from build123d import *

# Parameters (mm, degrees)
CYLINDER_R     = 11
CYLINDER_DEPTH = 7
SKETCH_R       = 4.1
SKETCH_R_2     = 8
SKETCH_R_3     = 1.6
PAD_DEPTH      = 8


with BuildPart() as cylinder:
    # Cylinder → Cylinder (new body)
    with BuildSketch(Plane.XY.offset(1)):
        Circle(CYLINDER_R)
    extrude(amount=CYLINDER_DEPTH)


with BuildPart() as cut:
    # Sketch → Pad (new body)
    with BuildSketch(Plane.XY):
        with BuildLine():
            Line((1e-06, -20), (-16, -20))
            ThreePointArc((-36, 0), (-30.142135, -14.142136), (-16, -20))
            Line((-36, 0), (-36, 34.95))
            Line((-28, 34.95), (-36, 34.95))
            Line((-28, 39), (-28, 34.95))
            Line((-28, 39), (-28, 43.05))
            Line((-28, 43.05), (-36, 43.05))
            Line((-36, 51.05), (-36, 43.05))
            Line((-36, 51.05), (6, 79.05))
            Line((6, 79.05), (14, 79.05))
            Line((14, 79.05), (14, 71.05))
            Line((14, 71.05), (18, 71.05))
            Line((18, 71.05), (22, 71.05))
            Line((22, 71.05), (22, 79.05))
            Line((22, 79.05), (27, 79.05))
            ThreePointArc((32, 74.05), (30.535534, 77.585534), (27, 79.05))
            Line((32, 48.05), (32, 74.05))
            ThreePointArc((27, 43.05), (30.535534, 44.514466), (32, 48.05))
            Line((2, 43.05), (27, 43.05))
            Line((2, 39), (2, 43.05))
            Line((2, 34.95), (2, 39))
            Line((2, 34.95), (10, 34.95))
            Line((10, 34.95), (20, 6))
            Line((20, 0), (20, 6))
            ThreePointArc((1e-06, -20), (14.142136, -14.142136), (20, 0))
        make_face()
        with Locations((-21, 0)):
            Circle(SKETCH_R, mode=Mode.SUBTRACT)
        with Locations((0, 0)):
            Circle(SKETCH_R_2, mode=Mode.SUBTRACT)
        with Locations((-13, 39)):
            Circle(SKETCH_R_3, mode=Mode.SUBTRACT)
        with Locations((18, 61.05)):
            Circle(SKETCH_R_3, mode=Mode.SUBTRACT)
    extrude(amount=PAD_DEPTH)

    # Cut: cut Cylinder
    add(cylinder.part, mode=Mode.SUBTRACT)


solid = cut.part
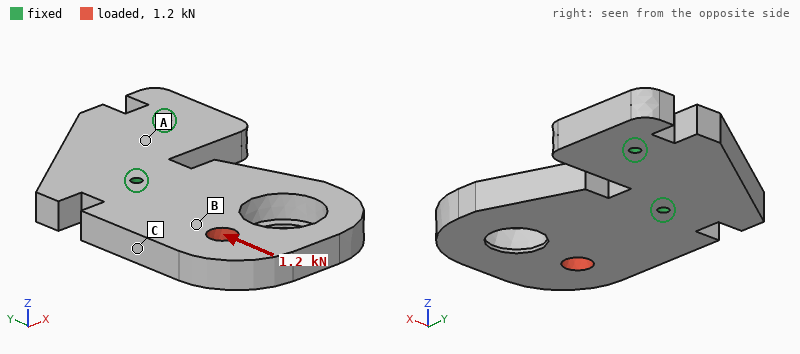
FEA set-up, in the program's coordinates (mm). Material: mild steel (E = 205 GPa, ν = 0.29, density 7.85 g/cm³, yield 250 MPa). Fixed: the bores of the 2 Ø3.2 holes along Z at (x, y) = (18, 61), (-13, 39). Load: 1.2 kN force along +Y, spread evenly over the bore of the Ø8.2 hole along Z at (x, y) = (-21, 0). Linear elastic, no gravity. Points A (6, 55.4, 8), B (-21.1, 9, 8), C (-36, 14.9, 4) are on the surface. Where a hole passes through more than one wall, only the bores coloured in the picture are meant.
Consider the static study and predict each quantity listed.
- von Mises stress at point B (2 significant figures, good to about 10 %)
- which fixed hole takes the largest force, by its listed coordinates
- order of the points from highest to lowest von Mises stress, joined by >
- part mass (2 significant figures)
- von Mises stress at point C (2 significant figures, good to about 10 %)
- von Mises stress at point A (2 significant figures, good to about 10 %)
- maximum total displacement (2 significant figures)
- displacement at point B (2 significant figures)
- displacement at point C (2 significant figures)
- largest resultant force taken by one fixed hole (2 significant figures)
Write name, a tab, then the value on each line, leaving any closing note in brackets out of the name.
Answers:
von Mises stress at point B	6.7 MPa
which fixed hole takes the largest force, by its listed coordinates	(-13, 39)
order of the points from highest to lowest von Mises stress, joined by >	B > C > A
part mass	270 g
von Mises stress at point C	4.1 MPa
von Mises stress at point A	2.0 MPa
maximum total displacement	5.5 µm
displacement at point B	3.1 µm
displacement at point C	3.7 µm
largest resultant force taken by one fixed hole	1.3 kN
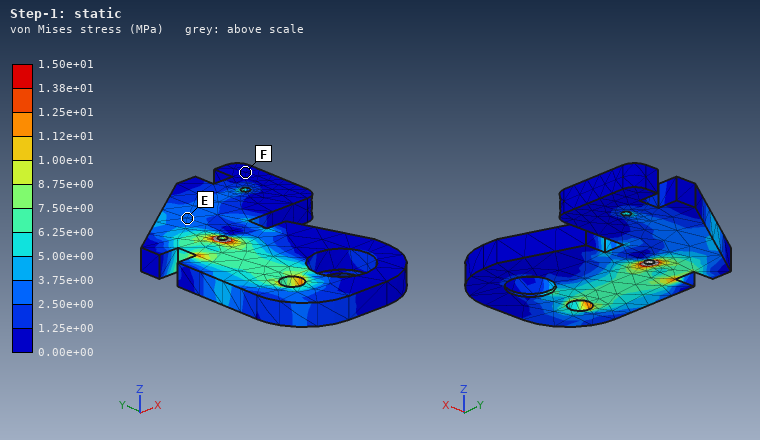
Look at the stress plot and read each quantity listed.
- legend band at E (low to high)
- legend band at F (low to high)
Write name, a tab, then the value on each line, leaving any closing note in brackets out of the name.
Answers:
legend band at E	2.50e+00 to 3.75e+00 MPa
legend band at F	0.00e+00 to 1.25e+00 MPa
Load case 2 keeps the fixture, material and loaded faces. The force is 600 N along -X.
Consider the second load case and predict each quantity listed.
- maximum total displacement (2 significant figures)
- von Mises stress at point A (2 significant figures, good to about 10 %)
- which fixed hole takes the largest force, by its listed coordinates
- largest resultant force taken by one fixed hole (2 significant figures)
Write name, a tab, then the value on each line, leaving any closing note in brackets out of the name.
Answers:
maximum total displacement	13 µm
von Mises stress at point A	5.5 MPa
which fixed hole takes the largest force, by its listed coordinates	(-13, 39)
largest resultant force taken by one fixed hole	1.1 kN
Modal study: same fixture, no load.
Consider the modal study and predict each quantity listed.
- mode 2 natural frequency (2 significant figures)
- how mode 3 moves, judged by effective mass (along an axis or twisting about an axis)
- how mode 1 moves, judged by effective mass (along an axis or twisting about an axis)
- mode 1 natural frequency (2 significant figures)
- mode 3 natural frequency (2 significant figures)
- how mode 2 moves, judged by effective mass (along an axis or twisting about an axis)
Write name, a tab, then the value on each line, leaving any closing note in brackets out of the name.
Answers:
mode 2 natural frequency	3300 Hz
how mode 3 moves, judged by effective mass	along X
how mode 1 moves, judged by effective mass	along Z
mode 1 natural frequency	1600 Hz
mode 3 natural frequency	3700 Hz
how mode 2 moves, judged by effective mass	twisting about Y
